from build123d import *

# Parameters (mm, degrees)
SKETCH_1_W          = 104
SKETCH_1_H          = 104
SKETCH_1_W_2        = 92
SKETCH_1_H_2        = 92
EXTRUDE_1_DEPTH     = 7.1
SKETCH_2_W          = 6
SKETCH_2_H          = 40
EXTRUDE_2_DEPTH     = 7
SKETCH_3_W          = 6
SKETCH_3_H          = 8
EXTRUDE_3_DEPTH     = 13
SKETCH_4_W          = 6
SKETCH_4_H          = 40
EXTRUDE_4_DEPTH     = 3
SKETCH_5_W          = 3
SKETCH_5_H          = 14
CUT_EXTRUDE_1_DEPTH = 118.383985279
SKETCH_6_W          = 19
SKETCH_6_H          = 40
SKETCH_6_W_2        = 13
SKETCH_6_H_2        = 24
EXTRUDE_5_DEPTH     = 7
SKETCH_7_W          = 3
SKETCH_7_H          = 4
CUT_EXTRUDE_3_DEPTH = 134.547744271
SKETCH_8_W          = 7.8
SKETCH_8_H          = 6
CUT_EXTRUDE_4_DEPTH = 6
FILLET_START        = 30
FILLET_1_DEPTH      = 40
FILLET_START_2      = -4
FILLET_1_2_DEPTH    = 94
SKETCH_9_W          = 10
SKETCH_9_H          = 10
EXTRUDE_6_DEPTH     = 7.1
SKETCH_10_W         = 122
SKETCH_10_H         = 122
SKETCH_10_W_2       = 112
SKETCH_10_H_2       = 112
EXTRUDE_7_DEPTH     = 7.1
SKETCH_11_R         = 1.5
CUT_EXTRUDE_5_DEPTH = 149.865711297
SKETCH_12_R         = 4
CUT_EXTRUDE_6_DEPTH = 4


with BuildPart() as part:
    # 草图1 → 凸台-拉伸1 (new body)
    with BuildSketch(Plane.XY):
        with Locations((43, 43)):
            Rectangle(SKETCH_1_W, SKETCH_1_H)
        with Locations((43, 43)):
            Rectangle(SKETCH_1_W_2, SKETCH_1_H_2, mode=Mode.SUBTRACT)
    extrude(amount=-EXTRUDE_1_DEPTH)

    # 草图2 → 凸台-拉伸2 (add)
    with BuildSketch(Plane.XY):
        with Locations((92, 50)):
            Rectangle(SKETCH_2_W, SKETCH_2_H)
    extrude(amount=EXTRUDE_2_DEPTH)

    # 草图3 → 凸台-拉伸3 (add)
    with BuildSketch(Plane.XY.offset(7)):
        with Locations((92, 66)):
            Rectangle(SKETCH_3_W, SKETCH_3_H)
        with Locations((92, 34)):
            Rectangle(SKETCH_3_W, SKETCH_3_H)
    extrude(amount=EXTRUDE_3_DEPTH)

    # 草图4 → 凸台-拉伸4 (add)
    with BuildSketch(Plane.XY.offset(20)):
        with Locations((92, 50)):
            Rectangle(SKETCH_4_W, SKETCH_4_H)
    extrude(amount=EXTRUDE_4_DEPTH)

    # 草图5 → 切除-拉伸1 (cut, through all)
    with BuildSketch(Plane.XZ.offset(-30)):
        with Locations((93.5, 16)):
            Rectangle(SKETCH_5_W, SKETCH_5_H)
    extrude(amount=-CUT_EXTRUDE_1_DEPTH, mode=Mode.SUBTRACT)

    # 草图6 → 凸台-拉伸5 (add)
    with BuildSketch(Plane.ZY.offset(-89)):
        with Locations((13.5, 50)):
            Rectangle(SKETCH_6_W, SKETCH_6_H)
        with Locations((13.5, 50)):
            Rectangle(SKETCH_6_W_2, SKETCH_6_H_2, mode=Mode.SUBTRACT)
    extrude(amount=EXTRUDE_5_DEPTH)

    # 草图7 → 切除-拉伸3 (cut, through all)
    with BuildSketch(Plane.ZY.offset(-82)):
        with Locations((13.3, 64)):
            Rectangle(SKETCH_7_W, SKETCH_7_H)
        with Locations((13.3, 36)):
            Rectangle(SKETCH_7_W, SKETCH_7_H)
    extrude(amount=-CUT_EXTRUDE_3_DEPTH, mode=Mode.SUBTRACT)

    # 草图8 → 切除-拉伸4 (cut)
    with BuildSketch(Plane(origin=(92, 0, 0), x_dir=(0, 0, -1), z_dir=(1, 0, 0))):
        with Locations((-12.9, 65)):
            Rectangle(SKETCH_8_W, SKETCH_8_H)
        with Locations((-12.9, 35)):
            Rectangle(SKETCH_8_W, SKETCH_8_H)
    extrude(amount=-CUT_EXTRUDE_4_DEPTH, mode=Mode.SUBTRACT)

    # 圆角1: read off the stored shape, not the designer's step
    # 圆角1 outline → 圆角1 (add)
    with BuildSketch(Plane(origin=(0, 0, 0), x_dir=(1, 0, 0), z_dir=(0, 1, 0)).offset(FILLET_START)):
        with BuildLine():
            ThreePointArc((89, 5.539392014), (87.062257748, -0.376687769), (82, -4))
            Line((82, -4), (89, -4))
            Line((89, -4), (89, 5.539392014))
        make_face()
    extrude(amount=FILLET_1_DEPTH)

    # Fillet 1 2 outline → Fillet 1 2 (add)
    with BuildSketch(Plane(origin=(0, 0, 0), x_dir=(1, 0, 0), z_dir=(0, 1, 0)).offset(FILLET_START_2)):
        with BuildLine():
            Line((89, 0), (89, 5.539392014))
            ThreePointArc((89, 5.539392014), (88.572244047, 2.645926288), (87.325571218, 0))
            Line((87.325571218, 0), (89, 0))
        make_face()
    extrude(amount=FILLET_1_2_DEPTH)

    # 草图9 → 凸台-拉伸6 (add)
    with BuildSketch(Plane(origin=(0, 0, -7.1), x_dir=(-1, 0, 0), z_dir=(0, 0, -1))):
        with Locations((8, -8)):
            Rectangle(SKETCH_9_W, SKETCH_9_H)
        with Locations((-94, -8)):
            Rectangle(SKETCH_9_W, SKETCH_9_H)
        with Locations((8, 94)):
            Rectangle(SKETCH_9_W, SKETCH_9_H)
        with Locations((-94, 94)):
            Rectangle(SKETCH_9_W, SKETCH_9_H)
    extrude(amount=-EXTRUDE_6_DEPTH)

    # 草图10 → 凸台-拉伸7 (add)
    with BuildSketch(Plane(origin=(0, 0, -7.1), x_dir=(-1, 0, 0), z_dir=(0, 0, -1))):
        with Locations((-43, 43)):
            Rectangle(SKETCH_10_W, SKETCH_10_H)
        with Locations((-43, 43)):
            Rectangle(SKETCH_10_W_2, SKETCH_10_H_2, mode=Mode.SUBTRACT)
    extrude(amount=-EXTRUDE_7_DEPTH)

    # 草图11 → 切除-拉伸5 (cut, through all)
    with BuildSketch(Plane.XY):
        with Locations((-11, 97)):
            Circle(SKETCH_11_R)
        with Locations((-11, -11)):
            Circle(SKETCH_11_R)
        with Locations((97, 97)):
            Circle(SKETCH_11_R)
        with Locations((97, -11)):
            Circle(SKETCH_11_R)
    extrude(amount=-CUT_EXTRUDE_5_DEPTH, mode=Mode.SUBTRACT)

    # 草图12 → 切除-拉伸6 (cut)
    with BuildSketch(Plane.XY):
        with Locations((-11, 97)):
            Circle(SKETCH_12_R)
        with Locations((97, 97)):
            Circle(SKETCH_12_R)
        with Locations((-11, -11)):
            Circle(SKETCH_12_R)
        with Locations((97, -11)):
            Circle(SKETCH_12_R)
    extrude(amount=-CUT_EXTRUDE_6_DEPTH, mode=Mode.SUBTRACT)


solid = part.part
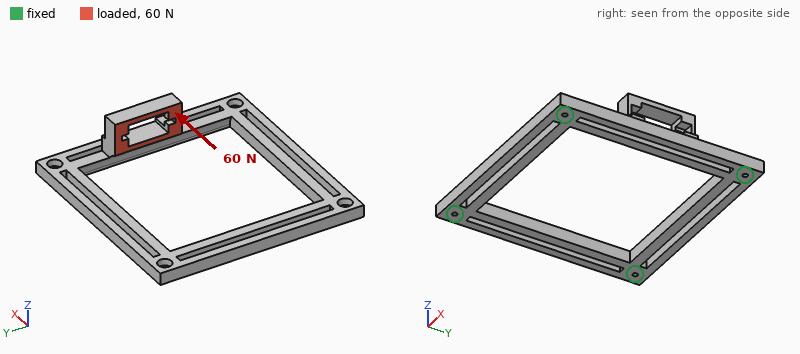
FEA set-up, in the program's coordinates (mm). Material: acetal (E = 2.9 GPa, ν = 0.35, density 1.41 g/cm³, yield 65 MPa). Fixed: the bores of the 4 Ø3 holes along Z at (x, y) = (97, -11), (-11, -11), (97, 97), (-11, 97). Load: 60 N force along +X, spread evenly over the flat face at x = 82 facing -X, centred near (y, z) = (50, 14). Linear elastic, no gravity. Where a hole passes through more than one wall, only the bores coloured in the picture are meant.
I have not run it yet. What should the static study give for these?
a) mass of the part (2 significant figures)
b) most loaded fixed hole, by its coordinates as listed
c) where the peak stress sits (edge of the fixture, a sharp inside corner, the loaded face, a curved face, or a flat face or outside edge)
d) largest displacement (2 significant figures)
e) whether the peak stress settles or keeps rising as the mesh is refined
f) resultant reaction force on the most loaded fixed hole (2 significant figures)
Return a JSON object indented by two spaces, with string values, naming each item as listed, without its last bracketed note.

{
  "mass of the part": "57 g",
  "most loaded fixed hole, by its coordinates as listed": "(-11, 97)",
  "where the peak stress sits": "edge of the fixture",
  "largest displacement": "2.0 mm",
  "whether the peak stress settles or keeps rising as the mesh is refined": "keeps rising",
  "resultant reaction force on the most loaded fixed hole": "32 N"
}
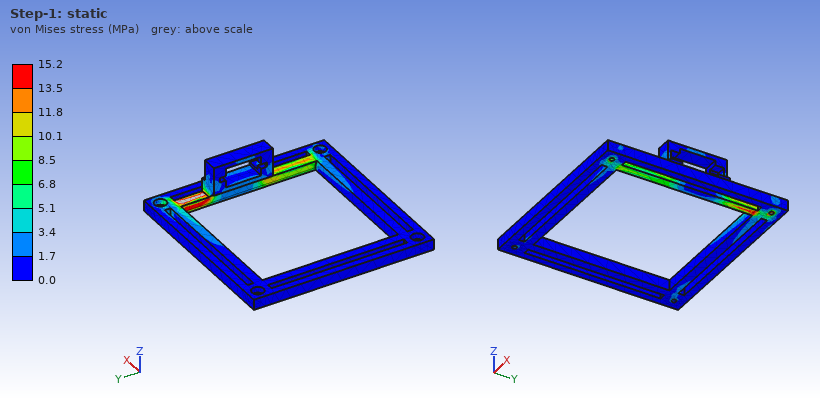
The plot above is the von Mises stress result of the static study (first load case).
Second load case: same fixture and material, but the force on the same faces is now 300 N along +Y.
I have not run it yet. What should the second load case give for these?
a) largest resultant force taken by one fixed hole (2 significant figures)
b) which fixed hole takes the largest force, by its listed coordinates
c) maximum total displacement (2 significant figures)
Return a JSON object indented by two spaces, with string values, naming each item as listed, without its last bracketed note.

{
  "largest resultant force taken by one fixed hole": "180 N",
  "which fixed hole takes the largest force, by its listed coordinates": "(97, -11)",
  "maximum total displacement": "1.0 mm"
}
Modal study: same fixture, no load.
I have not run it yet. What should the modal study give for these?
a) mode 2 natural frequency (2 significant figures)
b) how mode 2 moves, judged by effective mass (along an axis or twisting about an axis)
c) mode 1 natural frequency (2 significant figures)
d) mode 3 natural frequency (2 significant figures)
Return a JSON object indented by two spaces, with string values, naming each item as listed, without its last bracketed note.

{
  "mode 2 natural frequency": "600 Hz",
  "how mode 2 moves, judged by effective mass": "along Z",
  "mode 1 natural frequency": "380 Hz",
  "mode 3 natural frequency": "690 Hz"
}
